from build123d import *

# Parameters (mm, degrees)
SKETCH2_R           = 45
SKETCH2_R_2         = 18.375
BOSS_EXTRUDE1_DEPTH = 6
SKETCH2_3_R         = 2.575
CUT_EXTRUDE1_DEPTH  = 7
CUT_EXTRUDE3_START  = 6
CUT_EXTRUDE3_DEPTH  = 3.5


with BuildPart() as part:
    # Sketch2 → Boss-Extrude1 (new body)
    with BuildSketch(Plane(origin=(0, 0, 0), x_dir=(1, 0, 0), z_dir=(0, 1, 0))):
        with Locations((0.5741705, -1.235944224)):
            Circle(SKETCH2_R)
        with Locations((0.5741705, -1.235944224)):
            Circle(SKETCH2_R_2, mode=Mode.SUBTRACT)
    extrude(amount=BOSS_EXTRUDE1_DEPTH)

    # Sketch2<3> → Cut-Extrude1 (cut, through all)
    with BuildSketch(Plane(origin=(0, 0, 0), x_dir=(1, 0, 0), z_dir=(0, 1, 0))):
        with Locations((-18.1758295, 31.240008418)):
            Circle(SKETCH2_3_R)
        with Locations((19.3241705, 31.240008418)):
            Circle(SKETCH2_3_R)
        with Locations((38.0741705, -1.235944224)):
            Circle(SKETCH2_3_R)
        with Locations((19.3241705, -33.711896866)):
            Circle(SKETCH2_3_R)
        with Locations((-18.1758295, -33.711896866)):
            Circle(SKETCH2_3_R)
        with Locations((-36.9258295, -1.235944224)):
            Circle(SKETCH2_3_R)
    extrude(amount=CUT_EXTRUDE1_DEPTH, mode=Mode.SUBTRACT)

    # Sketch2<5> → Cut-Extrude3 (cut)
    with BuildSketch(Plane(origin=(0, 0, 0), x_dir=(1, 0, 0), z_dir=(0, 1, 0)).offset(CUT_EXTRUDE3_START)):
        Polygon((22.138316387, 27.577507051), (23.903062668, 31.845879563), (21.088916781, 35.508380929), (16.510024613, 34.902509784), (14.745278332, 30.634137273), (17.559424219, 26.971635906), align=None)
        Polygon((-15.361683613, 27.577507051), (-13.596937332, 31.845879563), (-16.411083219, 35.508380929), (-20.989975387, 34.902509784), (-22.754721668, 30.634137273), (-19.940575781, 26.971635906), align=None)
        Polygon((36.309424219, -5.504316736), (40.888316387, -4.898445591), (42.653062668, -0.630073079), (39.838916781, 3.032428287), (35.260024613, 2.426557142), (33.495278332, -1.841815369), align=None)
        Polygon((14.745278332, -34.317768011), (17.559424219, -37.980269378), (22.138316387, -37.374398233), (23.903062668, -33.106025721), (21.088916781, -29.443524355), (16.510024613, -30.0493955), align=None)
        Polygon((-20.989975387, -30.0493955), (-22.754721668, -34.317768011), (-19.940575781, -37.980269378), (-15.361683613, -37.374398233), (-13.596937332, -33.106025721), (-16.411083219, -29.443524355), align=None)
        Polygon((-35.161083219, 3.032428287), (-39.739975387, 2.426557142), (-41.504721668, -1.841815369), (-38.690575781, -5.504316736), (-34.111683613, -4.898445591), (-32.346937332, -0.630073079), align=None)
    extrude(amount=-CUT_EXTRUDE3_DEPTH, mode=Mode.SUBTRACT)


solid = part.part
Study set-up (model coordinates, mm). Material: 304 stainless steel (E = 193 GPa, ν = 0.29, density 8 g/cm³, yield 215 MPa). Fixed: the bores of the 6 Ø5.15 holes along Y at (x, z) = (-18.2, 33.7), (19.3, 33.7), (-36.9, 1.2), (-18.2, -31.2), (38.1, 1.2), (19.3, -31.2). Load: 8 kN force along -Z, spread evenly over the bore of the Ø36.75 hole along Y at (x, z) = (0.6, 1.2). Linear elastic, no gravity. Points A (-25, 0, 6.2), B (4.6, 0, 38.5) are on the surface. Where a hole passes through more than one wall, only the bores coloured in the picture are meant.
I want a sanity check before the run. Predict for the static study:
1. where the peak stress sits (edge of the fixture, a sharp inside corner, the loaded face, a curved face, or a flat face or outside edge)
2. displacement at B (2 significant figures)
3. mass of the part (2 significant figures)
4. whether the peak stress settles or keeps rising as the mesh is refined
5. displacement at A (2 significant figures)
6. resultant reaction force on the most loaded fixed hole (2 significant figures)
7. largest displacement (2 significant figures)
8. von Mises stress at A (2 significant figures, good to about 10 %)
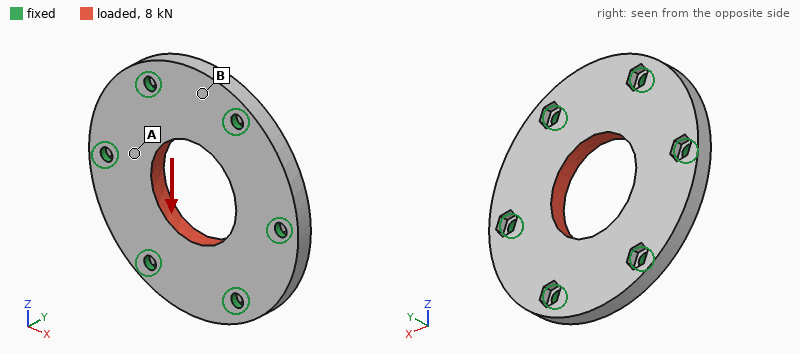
edge of the fixture
1.4 µm
240 g
keeps rising
1.6 µm
1.5 kN
4.0 µm
15 MPa
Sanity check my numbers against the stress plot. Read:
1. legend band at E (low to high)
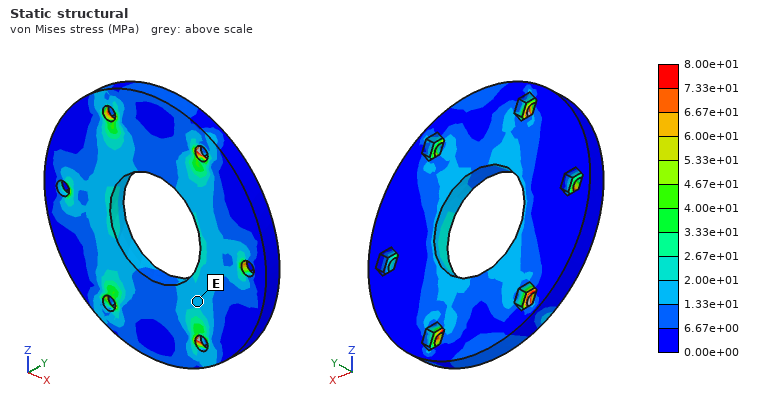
1.33e+01 to 2.00e+01 MPa
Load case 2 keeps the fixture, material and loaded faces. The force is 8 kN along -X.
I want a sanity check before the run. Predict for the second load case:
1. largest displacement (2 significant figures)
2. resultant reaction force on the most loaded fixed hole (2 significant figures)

3.8 µm
1.7 kN
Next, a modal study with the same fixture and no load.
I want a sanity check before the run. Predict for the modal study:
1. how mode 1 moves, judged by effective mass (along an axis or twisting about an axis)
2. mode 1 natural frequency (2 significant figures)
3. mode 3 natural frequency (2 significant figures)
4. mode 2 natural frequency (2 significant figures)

along Y
8900 Hz
12 kHz
12 kHz
